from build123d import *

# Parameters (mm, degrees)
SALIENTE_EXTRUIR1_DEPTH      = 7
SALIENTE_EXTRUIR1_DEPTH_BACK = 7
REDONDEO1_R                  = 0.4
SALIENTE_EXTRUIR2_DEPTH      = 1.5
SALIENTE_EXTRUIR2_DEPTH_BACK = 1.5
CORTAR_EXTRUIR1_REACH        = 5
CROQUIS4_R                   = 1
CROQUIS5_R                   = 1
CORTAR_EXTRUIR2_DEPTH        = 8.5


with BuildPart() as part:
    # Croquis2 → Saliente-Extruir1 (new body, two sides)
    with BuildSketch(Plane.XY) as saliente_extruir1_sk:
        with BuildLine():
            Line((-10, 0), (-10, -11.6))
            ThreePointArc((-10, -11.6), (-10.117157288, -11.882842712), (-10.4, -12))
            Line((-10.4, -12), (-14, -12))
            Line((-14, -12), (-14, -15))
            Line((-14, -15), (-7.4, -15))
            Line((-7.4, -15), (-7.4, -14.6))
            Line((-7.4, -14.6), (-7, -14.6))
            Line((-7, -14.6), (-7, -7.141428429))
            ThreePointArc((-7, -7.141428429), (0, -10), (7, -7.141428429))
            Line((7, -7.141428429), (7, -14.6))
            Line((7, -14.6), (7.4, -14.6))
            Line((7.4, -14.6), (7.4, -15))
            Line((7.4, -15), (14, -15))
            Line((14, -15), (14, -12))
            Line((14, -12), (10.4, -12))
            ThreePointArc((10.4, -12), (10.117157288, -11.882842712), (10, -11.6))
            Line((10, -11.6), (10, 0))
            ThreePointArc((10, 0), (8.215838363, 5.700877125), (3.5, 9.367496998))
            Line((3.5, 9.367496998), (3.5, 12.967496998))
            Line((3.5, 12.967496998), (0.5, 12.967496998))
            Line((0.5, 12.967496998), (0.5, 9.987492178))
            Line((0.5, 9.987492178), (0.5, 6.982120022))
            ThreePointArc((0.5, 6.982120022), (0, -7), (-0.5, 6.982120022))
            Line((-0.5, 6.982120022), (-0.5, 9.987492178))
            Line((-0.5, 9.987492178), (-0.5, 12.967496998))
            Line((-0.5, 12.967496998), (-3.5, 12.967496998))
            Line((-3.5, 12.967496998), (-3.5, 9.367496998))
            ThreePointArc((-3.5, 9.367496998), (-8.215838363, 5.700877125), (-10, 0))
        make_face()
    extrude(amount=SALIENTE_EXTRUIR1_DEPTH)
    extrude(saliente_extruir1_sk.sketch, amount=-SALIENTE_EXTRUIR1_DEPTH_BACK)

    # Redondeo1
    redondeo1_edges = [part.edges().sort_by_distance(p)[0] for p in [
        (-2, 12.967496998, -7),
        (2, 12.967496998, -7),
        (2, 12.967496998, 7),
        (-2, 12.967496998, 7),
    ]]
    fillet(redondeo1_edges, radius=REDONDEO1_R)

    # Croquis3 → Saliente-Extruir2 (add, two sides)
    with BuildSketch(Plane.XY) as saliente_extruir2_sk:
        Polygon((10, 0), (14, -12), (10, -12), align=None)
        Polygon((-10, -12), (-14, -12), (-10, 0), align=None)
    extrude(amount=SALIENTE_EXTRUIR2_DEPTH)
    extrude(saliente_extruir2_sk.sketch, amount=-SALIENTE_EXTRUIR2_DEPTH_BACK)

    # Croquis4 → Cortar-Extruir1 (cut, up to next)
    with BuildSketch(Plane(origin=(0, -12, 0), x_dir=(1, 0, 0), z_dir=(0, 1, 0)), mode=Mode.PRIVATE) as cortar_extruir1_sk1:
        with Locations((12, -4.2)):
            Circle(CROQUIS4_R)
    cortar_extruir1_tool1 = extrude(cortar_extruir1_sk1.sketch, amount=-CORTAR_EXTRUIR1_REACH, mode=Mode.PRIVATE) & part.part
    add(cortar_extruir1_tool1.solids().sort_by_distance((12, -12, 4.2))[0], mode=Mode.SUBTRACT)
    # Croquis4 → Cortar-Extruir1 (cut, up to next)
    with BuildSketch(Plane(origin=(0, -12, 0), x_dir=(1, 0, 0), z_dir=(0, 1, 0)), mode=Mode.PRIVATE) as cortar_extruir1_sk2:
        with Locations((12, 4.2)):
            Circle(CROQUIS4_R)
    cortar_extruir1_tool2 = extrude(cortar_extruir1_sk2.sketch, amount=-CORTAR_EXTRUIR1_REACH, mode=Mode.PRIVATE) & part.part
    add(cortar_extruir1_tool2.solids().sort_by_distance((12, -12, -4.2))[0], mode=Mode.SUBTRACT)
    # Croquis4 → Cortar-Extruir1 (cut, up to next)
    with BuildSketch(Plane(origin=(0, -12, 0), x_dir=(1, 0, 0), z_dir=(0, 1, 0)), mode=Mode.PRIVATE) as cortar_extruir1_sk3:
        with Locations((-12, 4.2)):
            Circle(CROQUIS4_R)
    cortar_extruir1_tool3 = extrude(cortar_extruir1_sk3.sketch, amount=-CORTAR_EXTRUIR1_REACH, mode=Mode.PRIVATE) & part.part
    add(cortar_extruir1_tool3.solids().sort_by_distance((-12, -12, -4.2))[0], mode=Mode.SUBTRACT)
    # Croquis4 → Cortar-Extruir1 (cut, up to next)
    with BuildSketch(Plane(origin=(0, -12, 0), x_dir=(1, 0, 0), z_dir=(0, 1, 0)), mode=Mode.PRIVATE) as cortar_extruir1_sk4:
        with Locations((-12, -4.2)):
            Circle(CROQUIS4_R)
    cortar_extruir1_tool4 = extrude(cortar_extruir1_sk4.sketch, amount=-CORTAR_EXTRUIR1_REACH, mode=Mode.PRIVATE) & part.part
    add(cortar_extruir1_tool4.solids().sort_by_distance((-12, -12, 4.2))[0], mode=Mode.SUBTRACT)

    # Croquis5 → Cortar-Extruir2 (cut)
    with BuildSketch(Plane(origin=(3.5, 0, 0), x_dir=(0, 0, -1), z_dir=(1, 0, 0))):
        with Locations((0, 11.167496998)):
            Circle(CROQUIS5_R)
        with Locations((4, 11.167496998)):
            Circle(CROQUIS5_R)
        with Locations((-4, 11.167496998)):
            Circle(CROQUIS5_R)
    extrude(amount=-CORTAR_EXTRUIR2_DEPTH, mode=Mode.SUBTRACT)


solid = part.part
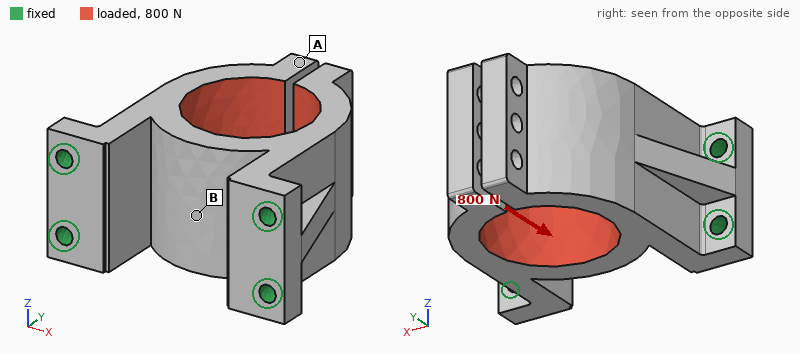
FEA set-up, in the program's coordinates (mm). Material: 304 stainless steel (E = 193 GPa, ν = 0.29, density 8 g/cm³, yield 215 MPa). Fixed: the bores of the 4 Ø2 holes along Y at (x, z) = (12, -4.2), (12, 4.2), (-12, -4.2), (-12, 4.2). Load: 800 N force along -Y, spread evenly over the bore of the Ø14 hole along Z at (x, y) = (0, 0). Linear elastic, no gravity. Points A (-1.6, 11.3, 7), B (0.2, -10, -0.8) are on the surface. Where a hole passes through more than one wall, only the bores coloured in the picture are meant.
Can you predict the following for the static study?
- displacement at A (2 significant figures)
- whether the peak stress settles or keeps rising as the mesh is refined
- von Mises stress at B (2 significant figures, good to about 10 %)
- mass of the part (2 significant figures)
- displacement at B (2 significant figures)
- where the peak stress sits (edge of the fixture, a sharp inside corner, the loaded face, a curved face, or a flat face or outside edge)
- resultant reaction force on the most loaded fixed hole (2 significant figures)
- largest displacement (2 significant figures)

23 µm
keeps rising
28 MPa
30 g
4.6 µm
edge of the fixture
240 N
26 µm
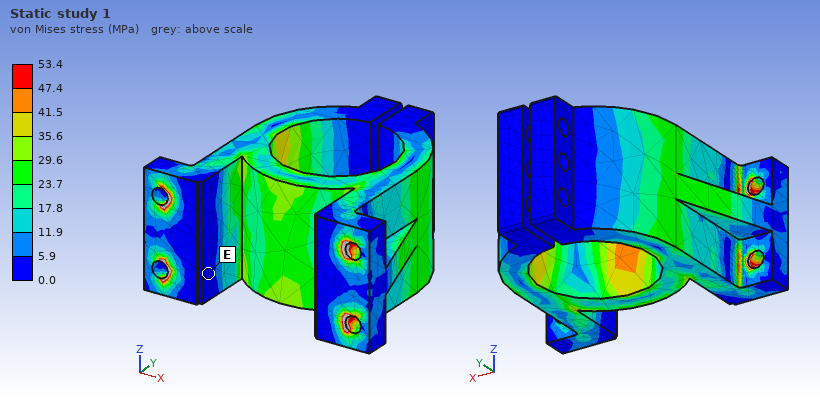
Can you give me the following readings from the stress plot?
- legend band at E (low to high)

0.0 to 5.9 MPa
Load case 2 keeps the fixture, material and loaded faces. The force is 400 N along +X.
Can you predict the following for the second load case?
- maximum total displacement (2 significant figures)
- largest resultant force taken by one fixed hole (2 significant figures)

18 µm
130 N
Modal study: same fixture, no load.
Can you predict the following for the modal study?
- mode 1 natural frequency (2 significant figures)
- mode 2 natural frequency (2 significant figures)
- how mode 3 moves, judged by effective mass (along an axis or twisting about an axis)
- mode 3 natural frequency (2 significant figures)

5500 Hz
5700 Hz
along Z
8300 Hz
